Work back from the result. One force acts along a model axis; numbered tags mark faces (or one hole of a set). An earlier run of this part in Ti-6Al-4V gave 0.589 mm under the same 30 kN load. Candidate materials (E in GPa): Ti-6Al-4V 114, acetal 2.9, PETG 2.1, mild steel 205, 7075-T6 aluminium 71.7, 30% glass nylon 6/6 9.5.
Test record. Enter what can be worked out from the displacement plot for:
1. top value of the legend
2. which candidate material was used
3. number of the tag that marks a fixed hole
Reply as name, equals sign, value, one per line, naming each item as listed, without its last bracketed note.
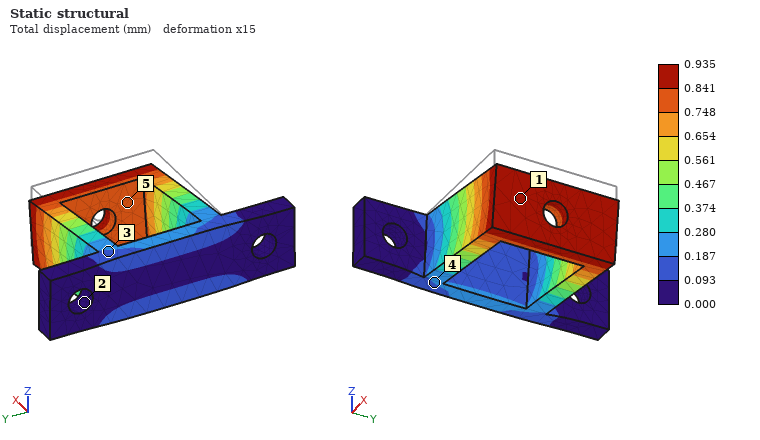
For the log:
top value of the legend = 0.935 mm
which candidate material was used = 7075-T6 aluminium
number of the tag that marks a fixed hole = 2
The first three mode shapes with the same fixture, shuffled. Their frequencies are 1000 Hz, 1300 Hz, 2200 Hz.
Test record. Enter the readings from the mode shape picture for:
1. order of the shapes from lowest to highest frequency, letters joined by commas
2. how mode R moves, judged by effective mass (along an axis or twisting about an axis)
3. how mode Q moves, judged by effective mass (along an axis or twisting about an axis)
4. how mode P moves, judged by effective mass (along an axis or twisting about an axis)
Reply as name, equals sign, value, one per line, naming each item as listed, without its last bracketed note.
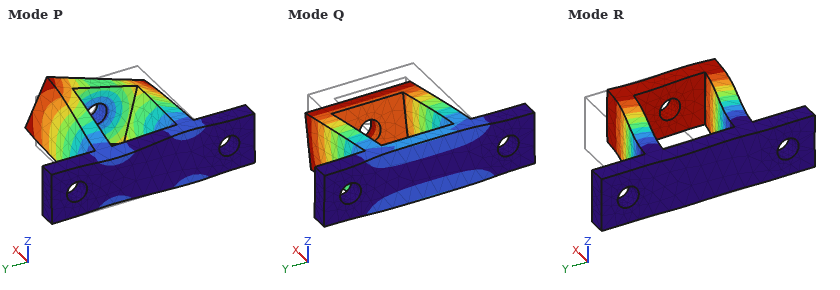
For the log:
order of the shapes from lowest to highest frequency, letters joined by commas = Q, R, P
how mode R moves, judged by effective mass = along Y
how mode Q moves, judged by effective mass = along Z
how mode P moves, judged by effective mass = twisting about X
